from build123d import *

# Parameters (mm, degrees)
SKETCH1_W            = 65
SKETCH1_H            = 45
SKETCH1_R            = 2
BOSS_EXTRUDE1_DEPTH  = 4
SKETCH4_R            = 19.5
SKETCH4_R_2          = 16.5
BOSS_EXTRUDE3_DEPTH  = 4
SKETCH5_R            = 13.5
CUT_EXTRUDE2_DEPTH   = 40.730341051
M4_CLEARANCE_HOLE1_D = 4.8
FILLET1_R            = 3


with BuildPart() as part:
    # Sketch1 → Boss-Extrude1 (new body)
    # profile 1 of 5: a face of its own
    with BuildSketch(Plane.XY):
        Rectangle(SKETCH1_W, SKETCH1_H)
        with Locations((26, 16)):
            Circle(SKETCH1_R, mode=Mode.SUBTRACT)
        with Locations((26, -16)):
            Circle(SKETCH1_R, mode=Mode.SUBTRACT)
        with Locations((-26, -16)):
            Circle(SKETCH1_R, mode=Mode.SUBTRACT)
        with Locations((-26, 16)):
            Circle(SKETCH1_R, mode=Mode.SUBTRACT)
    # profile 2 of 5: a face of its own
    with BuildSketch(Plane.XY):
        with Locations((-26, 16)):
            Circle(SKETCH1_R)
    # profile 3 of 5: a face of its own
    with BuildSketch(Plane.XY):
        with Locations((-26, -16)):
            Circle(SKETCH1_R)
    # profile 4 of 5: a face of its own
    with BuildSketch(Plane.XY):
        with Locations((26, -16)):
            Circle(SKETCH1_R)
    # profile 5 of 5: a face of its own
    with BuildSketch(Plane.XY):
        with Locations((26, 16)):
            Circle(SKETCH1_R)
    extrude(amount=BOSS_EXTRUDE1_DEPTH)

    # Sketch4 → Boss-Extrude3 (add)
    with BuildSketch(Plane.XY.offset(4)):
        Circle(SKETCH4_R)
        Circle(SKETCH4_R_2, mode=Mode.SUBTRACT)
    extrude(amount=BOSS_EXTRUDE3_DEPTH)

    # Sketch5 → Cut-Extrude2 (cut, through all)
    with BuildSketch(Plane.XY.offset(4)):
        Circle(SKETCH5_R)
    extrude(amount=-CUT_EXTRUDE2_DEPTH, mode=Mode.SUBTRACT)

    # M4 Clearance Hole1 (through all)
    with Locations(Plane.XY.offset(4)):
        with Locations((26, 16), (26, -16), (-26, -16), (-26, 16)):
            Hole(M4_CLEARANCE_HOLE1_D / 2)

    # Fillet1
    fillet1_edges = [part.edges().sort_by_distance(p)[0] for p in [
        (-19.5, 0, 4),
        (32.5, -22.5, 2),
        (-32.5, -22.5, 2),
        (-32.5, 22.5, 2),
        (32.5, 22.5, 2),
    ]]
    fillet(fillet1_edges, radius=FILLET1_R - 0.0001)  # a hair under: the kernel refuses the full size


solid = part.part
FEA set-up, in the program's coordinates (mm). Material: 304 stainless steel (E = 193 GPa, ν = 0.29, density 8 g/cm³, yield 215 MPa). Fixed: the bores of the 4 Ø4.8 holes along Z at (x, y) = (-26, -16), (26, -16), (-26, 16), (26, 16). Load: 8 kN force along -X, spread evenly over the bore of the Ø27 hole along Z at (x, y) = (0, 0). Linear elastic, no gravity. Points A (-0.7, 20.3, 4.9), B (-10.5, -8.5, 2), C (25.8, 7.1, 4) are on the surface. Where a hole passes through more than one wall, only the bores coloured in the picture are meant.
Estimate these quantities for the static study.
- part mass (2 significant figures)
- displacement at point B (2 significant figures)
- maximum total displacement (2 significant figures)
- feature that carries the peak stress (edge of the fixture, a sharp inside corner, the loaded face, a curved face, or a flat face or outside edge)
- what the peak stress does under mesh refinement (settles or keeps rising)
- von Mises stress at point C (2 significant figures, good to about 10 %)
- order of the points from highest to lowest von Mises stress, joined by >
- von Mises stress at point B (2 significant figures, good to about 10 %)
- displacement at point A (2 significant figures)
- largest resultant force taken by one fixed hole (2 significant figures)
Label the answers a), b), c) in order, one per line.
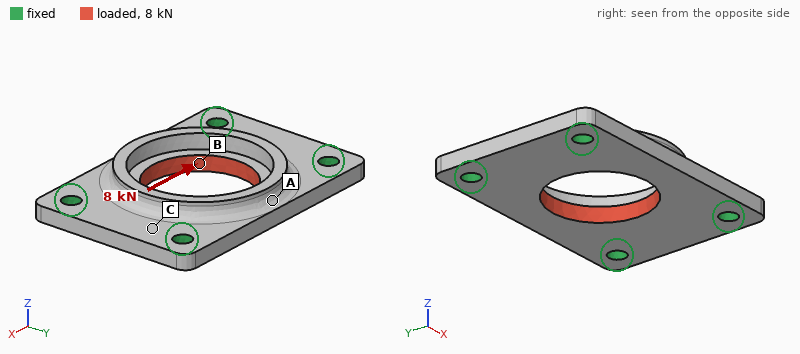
a) 86 g
b) 3.1 µm
c) 3.6 µm
d) edge of the fixture
e) keeps rising
f) 18 MPa
g) B > C > A
h) 32 MPa
i) 2.2 µm
j) 2.1 kN
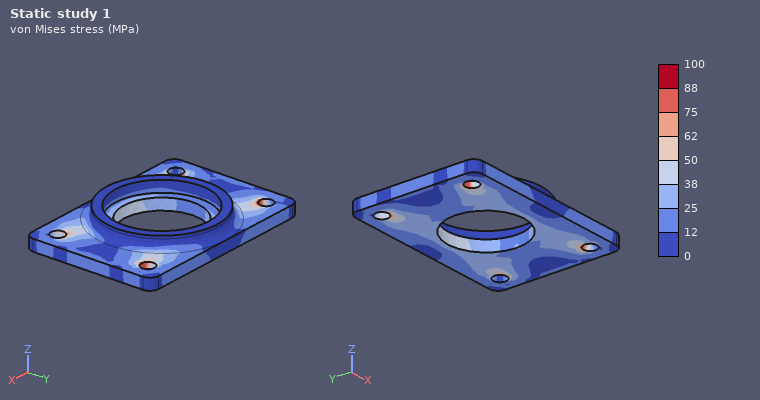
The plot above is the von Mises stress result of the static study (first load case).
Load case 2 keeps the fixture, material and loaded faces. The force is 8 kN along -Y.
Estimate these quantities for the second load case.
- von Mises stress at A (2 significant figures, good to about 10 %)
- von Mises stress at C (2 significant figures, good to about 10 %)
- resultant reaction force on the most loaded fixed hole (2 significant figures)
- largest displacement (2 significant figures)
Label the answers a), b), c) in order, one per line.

a) 35 MPa
b) 35 MPa
c) 2.2 kN
d) 11 µm
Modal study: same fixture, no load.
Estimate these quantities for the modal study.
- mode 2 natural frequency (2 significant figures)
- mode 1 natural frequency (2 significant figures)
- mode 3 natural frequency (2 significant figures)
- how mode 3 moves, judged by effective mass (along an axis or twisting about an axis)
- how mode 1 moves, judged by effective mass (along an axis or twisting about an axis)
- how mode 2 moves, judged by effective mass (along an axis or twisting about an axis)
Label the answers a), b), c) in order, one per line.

a) 10 kHz
b) 9100 Hz
c) 17 kHz
d) twisting about Y
e) along Z
f) twisting about X
